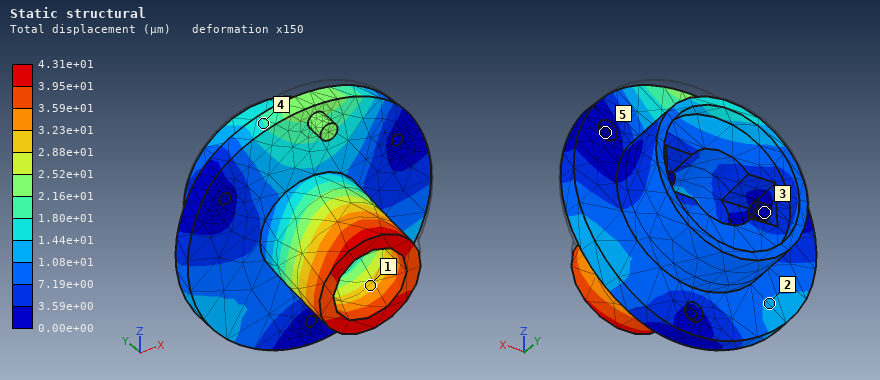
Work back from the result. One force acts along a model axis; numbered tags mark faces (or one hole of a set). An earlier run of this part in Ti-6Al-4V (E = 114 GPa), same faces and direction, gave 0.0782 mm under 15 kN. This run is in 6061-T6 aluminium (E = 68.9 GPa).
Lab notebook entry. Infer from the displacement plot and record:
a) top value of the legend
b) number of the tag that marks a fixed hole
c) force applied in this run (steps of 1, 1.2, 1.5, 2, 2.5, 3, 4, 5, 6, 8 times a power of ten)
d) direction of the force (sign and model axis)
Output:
4.31e+01 µm
5
5 kN
-Z
